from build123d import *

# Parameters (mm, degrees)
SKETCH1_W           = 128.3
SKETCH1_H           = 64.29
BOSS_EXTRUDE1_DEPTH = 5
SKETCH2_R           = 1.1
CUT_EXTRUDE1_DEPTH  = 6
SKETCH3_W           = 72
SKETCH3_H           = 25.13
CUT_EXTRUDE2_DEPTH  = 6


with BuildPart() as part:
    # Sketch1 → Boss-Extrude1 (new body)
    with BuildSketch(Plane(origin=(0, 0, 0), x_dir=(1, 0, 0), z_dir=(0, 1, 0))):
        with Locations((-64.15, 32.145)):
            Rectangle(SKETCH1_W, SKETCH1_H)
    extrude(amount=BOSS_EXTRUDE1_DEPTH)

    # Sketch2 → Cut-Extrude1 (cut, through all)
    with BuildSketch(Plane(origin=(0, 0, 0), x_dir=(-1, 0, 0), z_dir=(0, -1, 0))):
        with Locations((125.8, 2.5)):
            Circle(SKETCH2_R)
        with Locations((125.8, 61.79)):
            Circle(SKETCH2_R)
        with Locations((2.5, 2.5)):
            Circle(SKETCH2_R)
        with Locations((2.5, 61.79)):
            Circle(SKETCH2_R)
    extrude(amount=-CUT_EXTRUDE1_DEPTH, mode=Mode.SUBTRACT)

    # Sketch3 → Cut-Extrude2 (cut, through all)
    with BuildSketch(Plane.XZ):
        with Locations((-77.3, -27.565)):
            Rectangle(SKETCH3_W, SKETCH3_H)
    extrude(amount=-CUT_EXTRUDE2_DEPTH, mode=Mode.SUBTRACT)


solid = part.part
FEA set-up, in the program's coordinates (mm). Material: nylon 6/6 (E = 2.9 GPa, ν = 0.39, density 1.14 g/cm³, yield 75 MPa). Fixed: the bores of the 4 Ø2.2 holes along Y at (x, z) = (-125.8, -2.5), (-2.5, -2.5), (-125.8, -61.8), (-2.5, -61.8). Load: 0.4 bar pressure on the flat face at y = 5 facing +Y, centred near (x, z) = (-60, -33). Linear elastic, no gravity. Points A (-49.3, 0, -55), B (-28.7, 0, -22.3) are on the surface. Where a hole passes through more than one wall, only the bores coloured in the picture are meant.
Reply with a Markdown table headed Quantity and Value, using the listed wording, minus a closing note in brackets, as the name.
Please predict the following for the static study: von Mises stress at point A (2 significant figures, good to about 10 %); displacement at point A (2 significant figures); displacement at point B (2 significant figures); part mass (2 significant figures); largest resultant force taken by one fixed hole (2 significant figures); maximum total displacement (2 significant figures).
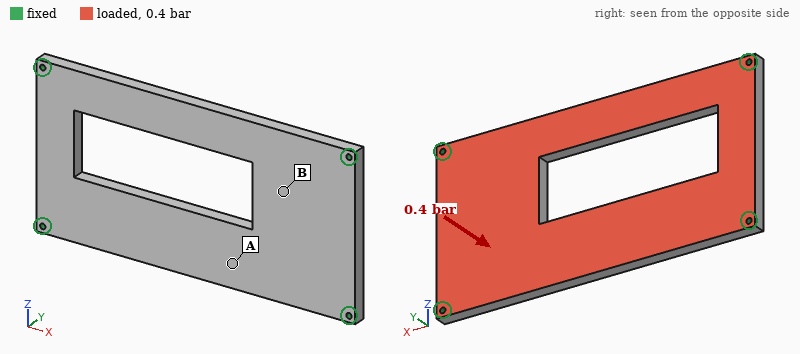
| Quantity | Value |
|---|---|
| von Mises stress at point A | 7.1 MPa |
| displacement at point A | 1.2 mm |
| displacement at point B | 0.77 mm |
| part mass | 37 g |
| largest resultant force taken by one fixed hole | 71 N |
| maximum total displacement | 1.4 mm |
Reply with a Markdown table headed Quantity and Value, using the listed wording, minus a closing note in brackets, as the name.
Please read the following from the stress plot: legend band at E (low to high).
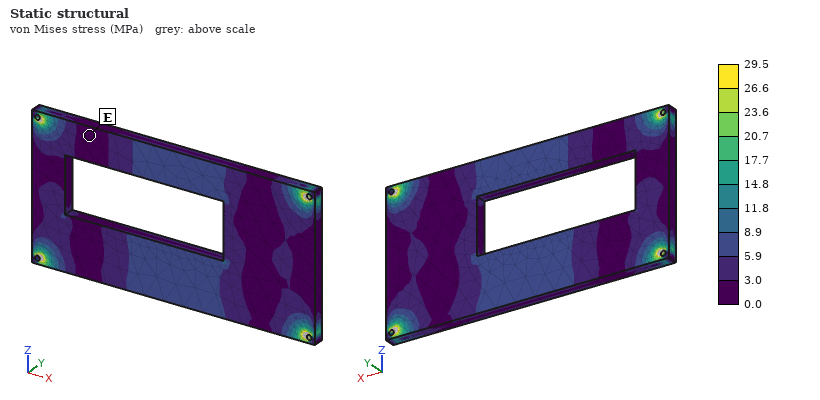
| Quantity | Value |
|---|---|
| legend band at E | 0.0 to 3.0 MPa |
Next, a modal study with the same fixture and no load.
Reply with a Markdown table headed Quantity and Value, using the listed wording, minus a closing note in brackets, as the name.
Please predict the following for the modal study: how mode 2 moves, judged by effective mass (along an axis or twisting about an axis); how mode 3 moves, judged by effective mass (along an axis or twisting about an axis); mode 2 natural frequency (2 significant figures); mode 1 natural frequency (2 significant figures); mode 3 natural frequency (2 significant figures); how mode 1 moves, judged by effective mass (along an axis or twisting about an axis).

| Quantity | Value |
|---|---|
| how mode 2 moves, judged by effective mass | twisting about X |
| how mode 3 moves, judged by effective mass | twisting about Z |
| mode 2 natural frequency | 650 Hz |
| mode 1 natural frequency | 420 Hz |
| mode 3 natural frequency | 1100 Hz |
| how mode 1 moves, judged by effective mass | along Y |
